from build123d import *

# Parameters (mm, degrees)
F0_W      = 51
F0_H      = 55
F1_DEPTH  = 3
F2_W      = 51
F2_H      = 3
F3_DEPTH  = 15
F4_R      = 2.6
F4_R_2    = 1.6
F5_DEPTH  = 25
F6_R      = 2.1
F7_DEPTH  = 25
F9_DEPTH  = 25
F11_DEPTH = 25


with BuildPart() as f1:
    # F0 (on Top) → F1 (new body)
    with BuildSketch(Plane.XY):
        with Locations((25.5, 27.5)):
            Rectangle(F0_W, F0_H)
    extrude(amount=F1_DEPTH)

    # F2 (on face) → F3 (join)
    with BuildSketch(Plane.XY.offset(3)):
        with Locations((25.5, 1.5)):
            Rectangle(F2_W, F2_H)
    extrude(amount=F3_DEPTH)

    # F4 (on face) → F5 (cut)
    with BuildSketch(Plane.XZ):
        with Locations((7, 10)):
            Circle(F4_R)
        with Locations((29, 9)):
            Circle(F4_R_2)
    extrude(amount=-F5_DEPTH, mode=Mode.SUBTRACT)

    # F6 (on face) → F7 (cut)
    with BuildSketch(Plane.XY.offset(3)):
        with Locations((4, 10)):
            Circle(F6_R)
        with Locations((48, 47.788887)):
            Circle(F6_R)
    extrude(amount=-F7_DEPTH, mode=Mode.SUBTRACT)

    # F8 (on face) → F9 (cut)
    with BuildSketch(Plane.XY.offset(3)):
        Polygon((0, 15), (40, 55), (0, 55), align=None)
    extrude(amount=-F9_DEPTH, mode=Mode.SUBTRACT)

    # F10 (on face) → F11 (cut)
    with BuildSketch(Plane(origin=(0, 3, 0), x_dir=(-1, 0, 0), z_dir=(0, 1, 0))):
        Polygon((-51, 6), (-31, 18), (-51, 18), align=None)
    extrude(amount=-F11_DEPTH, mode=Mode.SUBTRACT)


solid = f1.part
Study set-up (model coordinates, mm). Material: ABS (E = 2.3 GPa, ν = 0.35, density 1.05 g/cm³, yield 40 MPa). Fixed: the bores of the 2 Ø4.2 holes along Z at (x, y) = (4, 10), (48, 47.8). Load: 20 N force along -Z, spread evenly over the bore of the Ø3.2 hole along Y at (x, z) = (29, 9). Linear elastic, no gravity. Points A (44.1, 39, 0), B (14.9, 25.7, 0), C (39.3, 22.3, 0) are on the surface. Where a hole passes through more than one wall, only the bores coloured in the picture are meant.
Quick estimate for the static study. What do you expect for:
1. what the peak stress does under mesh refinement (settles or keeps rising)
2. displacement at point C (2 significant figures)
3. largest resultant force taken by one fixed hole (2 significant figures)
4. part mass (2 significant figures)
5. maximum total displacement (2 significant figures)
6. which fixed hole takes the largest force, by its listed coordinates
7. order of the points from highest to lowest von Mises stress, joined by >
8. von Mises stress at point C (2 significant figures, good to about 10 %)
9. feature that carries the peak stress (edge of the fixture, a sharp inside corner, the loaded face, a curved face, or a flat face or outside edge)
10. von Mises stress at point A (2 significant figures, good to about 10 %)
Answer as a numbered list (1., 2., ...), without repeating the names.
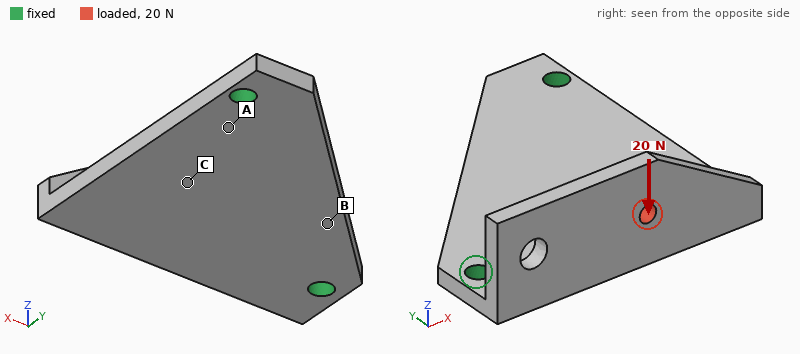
1. keeps rising
2. 0.25 mm
3. 17 N
4. 8.2 g
5. 0.86 mm
6. (4, 10)
7. A > C > B
8. 2.0 MPa
9. edge of the fixture
10. 3.3 MPa
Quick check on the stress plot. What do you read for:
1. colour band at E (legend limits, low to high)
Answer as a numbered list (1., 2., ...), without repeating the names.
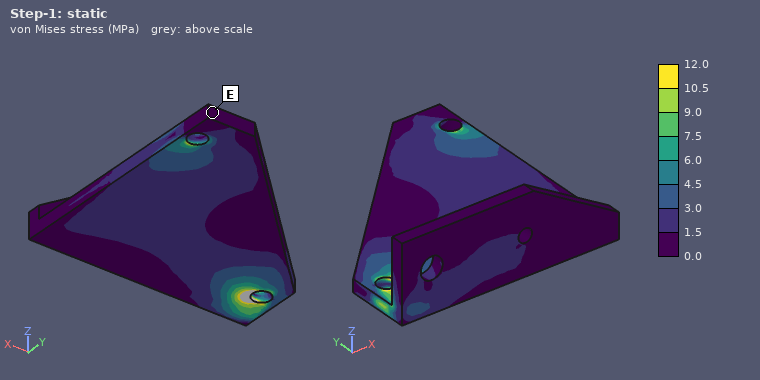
1. 0.0 to 1.5 MPa
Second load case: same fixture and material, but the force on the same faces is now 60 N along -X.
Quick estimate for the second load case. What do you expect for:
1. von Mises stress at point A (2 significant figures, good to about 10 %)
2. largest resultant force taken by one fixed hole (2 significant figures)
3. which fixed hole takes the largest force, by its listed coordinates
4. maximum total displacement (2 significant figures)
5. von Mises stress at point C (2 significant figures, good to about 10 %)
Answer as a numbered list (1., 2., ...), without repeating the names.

1. 3.2 MPa
2. 57 N
3. (4, 10)
4. 0.77 mm
5. 1.8 MPa
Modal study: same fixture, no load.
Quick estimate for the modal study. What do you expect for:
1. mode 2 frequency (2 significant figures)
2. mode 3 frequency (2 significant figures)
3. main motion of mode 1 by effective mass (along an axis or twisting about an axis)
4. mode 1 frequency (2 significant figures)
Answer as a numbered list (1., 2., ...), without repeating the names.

1. 1300 Hz
2. 1800 Hz
3. along Z
4. 510 Hz
